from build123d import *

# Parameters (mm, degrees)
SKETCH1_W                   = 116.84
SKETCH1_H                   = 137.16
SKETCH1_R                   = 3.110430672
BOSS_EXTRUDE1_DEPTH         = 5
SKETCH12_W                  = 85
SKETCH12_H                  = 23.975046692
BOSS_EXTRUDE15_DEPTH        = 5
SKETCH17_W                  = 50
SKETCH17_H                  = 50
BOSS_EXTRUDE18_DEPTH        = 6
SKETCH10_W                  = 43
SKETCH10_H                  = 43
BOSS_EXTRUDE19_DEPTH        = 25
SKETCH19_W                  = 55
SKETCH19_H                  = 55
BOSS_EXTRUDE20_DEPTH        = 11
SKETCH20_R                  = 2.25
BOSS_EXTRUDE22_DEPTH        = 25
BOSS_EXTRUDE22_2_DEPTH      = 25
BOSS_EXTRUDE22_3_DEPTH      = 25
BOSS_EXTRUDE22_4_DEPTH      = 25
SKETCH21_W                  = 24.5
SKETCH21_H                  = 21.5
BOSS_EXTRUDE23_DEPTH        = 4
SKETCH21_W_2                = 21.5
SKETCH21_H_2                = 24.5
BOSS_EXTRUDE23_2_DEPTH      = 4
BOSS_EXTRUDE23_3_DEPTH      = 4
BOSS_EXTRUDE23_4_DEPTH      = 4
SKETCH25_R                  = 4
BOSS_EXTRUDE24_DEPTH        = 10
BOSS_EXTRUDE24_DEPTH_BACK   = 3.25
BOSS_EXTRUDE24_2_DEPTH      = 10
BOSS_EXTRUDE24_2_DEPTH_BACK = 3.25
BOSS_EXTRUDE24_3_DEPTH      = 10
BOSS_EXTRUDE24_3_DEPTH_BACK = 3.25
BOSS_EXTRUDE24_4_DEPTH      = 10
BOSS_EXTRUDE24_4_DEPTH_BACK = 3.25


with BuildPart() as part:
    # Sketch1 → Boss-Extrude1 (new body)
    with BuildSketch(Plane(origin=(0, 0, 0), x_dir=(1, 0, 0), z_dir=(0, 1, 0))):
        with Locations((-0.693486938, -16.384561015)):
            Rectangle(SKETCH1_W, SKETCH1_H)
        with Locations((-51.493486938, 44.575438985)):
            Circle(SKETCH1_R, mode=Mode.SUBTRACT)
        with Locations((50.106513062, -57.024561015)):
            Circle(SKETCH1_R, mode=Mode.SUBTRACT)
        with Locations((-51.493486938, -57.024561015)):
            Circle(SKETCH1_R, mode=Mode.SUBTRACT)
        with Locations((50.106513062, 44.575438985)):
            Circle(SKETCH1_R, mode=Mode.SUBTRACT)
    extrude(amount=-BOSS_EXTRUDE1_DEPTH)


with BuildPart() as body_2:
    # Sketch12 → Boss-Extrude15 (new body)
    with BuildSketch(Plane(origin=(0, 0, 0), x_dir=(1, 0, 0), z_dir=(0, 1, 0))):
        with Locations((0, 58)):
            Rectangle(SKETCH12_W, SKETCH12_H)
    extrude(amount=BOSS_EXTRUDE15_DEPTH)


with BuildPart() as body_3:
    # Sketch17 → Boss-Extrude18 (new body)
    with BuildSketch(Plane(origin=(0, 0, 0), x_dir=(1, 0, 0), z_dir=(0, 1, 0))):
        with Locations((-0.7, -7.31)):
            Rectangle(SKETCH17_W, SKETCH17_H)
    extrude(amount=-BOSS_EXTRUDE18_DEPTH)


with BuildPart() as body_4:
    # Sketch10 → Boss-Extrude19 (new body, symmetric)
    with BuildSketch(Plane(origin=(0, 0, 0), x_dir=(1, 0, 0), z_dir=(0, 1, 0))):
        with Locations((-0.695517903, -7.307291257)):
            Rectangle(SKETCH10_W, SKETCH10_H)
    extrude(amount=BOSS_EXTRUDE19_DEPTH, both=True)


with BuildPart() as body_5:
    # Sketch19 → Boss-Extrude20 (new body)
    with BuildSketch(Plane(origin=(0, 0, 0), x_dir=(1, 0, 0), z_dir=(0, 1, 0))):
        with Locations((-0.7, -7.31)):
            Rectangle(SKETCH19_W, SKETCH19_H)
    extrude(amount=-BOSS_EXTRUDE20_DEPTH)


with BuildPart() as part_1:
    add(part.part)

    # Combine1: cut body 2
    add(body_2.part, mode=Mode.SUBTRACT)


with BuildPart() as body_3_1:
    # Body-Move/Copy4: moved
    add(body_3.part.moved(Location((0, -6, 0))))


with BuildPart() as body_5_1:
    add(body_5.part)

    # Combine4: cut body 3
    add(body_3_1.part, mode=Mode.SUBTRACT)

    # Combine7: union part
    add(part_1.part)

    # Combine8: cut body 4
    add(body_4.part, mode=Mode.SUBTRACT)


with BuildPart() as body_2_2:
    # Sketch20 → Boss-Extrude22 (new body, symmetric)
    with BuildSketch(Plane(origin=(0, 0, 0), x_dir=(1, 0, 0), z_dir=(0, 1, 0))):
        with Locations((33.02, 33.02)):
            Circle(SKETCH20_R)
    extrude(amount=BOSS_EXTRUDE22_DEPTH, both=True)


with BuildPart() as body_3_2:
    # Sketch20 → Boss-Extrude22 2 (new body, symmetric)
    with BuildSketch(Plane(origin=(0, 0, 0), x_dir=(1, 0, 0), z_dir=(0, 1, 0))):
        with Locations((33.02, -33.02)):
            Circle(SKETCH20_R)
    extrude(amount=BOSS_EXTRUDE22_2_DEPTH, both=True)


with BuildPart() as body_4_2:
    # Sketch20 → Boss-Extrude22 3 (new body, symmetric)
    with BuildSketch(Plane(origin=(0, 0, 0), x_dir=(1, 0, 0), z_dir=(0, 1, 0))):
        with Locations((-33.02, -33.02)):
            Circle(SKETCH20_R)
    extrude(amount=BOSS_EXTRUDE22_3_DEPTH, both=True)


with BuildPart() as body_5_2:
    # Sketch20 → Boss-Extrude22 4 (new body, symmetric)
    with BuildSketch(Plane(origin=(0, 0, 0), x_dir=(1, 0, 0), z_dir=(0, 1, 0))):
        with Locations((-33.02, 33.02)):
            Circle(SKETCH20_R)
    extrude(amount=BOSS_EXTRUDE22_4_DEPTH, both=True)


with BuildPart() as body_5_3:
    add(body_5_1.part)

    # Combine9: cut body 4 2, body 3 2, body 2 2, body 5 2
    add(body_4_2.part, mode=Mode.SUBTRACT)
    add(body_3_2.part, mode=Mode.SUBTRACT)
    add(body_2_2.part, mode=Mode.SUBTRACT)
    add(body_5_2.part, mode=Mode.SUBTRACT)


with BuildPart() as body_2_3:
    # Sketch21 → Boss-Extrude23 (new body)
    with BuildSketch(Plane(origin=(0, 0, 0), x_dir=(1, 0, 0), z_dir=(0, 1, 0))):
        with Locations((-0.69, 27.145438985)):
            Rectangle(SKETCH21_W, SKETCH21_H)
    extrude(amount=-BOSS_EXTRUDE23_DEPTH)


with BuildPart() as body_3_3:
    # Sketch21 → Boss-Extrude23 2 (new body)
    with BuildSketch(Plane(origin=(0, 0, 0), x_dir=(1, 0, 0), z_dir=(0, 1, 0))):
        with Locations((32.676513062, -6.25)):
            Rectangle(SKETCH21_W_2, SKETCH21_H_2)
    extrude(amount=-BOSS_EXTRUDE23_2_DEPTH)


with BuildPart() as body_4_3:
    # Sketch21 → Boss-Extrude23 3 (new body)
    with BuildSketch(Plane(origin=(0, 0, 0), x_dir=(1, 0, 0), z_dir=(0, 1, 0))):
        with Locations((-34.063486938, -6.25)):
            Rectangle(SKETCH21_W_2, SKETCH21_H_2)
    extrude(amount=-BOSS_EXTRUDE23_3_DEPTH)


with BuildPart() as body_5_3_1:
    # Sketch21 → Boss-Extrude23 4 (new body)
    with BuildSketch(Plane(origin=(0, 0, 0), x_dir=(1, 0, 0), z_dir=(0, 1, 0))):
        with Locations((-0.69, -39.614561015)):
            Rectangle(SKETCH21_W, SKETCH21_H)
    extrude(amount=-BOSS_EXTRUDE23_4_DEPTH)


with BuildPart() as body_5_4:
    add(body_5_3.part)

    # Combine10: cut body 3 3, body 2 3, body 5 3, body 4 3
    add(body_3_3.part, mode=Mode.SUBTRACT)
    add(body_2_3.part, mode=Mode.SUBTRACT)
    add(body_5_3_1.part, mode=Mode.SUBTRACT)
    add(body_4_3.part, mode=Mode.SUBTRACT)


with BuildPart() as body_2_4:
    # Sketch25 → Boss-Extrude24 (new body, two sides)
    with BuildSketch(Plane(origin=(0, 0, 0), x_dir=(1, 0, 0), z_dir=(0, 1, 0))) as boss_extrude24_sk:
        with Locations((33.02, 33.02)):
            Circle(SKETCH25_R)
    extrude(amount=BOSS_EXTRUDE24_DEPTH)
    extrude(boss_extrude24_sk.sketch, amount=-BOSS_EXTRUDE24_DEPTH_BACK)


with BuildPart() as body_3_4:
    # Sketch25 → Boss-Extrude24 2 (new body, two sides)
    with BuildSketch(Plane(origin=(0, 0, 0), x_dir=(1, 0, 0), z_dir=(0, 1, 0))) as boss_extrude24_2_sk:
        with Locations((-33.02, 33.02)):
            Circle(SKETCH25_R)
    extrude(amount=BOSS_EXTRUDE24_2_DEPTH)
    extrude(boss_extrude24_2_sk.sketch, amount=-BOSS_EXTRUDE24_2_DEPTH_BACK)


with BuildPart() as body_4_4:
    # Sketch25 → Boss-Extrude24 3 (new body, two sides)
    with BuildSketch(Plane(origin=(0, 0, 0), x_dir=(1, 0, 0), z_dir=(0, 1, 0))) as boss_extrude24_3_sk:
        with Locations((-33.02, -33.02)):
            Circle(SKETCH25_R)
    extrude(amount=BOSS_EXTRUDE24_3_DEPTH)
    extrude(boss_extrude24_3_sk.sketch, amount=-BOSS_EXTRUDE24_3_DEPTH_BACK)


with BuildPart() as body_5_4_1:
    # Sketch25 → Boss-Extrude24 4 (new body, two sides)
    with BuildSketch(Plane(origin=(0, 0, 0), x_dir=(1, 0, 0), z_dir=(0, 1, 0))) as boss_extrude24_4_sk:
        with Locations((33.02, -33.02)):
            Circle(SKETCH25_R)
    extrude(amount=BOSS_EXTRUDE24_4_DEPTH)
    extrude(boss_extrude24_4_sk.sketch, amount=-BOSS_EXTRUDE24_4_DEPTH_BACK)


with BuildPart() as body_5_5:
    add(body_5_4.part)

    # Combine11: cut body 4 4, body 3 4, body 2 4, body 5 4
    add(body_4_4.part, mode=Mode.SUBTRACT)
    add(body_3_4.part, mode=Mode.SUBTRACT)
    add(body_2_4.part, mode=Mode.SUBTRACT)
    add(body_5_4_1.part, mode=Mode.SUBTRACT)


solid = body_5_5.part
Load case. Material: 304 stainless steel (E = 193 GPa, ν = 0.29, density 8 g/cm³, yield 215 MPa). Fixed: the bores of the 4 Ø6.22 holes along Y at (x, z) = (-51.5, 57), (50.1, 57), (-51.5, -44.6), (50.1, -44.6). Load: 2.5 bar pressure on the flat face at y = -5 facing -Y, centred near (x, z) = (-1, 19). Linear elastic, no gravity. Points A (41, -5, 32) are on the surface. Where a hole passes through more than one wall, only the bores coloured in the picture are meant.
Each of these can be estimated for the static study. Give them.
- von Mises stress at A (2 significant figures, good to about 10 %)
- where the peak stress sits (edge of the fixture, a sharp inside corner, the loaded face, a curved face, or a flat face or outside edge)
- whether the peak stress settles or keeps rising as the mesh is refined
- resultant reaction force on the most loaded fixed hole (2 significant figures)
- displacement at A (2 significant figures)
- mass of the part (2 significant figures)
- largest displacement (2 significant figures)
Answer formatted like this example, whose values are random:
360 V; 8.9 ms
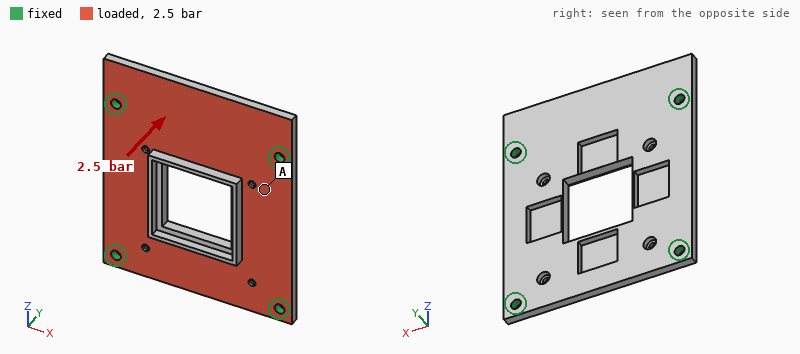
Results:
13 MPa; edge of the fixture; keeps rising; 1.1 kN; 24 µm; 520 g; 50 µm
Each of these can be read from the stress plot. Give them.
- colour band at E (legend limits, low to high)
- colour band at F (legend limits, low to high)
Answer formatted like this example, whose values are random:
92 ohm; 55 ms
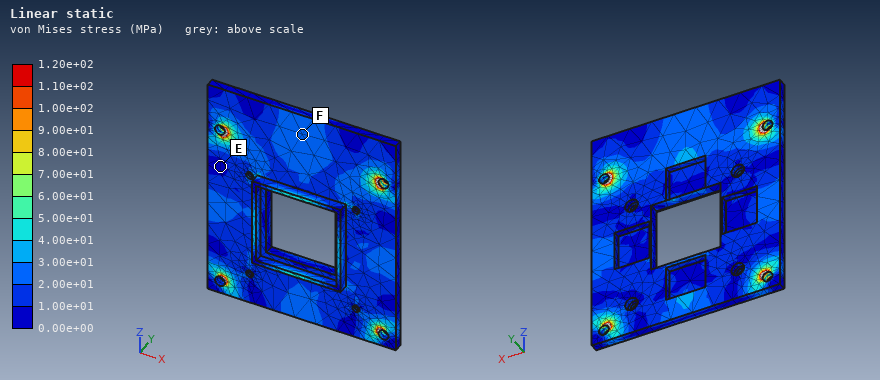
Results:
0.00e+00 to 1.00e+01 MPa; 2.00e+01 to 3.00e+01 MPa
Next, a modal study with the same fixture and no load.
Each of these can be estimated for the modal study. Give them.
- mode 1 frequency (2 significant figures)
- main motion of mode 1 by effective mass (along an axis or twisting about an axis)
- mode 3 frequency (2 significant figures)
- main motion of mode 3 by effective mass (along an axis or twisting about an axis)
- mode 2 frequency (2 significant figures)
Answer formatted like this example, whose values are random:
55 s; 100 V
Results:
2100 Hz; along Y; 2800 Hz; twisting about Z; 2200 Hz
